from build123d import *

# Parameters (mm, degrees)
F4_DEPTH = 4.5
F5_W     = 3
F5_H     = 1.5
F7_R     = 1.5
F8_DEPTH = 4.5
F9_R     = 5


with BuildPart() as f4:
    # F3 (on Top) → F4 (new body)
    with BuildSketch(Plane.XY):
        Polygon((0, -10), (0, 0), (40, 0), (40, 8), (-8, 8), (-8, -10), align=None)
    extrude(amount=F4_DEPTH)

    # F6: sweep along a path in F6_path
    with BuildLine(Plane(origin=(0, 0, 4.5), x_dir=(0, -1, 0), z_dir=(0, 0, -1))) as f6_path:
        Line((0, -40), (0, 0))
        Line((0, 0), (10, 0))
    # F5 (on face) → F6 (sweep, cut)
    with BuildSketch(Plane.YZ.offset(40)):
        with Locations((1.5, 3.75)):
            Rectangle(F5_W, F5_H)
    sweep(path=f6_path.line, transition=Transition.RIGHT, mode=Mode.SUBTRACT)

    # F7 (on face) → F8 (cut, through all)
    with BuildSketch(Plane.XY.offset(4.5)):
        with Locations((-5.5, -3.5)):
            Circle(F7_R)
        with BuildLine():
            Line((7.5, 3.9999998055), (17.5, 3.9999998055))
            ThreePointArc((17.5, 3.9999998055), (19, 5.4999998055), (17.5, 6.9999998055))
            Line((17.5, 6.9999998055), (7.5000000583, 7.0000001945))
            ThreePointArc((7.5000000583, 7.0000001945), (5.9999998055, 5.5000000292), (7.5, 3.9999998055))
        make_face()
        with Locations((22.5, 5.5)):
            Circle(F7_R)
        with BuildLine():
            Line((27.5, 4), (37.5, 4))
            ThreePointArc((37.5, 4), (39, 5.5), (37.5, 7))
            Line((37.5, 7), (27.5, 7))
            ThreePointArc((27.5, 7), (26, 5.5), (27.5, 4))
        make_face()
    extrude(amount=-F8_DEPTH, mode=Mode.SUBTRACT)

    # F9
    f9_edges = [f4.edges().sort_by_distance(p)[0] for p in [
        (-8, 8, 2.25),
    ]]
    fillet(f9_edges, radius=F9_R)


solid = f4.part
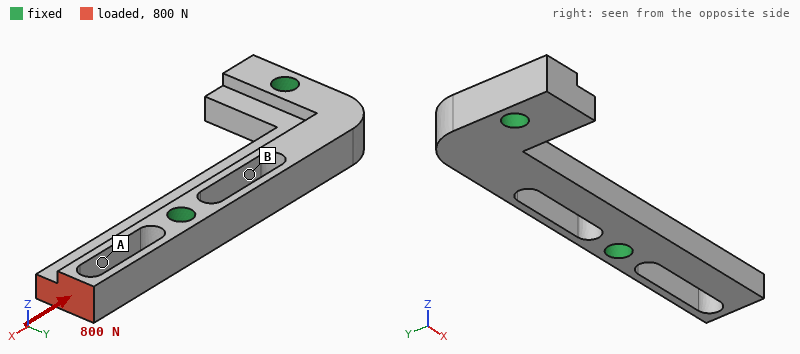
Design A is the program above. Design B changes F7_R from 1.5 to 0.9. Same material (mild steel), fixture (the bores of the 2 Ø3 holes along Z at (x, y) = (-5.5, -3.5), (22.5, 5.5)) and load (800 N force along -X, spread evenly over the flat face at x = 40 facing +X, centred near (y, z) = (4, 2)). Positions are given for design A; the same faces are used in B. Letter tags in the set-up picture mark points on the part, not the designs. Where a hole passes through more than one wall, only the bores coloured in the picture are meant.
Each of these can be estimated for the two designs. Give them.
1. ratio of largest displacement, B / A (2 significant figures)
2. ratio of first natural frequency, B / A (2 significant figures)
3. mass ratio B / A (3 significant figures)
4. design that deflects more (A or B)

0.91
0.94
1.03
A
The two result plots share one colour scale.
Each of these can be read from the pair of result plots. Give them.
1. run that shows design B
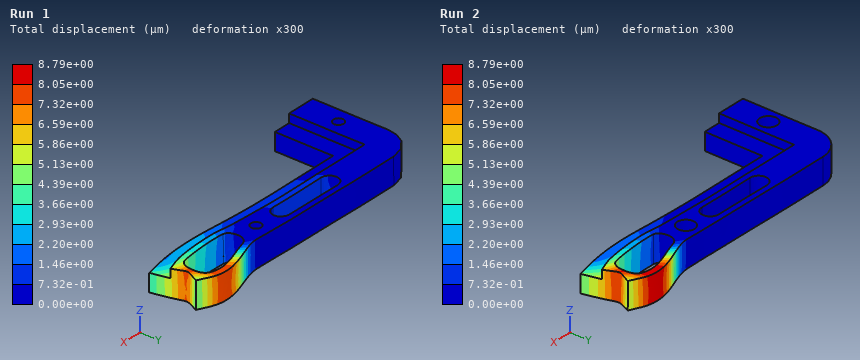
Run 1
